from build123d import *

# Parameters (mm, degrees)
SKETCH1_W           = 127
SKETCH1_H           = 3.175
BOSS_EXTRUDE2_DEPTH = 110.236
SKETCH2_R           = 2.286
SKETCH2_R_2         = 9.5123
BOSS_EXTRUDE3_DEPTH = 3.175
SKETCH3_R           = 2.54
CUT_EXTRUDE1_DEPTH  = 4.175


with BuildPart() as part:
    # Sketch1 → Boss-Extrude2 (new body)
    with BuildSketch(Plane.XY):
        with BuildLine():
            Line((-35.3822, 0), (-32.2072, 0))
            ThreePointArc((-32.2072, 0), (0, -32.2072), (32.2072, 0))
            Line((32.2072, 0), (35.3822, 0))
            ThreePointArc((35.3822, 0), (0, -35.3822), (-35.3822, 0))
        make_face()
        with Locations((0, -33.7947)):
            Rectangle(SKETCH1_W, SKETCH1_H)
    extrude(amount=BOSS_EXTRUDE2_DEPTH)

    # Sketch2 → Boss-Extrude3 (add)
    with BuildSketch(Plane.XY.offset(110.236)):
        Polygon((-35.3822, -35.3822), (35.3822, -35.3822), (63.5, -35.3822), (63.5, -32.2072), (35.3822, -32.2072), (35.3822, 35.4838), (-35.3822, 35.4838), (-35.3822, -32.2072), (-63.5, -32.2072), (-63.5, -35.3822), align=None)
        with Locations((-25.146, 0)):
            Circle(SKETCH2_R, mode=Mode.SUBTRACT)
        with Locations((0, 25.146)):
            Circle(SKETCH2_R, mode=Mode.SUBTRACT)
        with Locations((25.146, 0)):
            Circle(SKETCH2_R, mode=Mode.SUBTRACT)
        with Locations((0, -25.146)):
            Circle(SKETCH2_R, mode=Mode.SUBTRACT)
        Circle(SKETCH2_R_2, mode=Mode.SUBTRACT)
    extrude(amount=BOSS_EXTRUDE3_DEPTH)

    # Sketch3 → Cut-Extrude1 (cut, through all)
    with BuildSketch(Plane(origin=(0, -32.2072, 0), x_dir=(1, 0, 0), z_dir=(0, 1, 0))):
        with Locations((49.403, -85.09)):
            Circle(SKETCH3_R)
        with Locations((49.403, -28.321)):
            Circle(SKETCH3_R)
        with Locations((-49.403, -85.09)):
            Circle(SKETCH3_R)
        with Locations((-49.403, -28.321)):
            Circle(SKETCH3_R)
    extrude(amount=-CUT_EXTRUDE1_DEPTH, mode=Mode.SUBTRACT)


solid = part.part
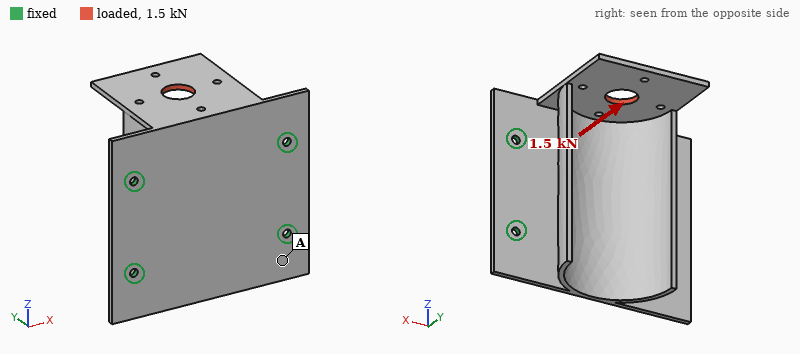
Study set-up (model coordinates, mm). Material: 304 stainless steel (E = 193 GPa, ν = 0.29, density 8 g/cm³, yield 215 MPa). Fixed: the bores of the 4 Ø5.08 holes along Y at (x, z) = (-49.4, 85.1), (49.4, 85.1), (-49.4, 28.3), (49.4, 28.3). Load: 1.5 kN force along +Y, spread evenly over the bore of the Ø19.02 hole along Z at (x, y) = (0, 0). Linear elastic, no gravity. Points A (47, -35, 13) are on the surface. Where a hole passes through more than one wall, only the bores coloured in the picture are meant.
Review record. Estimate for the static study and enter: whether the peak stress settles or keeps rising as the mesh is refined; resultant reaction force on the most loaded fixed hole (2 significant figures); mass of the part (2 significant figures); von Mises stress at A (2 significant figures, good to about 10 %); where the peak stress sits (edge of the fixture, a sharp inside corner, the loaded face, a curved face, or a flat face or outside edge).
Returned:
keeps rising
1.0 kN
720 g
25 MPa
edge of the fixture
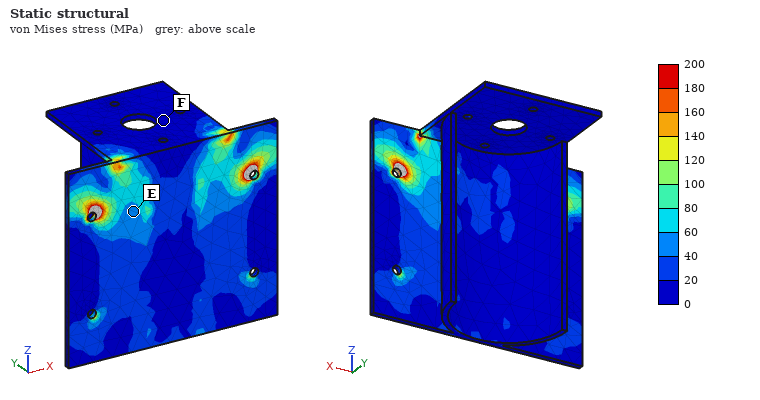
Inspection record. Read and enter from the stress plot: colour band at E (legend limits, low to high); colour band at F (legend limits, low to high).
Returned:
40 to 60 MPa
0 to 20 MPa
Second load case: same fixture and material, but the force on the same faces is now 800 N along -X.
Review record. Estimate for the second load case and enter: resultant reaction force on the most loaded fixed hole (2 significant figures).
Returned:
530 N
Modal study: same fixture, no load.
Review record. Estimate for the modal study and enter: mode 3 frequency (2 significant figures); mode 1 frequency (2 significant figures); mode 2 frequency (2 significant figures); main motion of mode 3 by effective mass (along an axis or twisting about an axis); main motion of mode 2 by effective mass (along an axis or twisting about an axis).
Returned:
1100 Hz
780 Hz
1100 Hz
along X
along Y
